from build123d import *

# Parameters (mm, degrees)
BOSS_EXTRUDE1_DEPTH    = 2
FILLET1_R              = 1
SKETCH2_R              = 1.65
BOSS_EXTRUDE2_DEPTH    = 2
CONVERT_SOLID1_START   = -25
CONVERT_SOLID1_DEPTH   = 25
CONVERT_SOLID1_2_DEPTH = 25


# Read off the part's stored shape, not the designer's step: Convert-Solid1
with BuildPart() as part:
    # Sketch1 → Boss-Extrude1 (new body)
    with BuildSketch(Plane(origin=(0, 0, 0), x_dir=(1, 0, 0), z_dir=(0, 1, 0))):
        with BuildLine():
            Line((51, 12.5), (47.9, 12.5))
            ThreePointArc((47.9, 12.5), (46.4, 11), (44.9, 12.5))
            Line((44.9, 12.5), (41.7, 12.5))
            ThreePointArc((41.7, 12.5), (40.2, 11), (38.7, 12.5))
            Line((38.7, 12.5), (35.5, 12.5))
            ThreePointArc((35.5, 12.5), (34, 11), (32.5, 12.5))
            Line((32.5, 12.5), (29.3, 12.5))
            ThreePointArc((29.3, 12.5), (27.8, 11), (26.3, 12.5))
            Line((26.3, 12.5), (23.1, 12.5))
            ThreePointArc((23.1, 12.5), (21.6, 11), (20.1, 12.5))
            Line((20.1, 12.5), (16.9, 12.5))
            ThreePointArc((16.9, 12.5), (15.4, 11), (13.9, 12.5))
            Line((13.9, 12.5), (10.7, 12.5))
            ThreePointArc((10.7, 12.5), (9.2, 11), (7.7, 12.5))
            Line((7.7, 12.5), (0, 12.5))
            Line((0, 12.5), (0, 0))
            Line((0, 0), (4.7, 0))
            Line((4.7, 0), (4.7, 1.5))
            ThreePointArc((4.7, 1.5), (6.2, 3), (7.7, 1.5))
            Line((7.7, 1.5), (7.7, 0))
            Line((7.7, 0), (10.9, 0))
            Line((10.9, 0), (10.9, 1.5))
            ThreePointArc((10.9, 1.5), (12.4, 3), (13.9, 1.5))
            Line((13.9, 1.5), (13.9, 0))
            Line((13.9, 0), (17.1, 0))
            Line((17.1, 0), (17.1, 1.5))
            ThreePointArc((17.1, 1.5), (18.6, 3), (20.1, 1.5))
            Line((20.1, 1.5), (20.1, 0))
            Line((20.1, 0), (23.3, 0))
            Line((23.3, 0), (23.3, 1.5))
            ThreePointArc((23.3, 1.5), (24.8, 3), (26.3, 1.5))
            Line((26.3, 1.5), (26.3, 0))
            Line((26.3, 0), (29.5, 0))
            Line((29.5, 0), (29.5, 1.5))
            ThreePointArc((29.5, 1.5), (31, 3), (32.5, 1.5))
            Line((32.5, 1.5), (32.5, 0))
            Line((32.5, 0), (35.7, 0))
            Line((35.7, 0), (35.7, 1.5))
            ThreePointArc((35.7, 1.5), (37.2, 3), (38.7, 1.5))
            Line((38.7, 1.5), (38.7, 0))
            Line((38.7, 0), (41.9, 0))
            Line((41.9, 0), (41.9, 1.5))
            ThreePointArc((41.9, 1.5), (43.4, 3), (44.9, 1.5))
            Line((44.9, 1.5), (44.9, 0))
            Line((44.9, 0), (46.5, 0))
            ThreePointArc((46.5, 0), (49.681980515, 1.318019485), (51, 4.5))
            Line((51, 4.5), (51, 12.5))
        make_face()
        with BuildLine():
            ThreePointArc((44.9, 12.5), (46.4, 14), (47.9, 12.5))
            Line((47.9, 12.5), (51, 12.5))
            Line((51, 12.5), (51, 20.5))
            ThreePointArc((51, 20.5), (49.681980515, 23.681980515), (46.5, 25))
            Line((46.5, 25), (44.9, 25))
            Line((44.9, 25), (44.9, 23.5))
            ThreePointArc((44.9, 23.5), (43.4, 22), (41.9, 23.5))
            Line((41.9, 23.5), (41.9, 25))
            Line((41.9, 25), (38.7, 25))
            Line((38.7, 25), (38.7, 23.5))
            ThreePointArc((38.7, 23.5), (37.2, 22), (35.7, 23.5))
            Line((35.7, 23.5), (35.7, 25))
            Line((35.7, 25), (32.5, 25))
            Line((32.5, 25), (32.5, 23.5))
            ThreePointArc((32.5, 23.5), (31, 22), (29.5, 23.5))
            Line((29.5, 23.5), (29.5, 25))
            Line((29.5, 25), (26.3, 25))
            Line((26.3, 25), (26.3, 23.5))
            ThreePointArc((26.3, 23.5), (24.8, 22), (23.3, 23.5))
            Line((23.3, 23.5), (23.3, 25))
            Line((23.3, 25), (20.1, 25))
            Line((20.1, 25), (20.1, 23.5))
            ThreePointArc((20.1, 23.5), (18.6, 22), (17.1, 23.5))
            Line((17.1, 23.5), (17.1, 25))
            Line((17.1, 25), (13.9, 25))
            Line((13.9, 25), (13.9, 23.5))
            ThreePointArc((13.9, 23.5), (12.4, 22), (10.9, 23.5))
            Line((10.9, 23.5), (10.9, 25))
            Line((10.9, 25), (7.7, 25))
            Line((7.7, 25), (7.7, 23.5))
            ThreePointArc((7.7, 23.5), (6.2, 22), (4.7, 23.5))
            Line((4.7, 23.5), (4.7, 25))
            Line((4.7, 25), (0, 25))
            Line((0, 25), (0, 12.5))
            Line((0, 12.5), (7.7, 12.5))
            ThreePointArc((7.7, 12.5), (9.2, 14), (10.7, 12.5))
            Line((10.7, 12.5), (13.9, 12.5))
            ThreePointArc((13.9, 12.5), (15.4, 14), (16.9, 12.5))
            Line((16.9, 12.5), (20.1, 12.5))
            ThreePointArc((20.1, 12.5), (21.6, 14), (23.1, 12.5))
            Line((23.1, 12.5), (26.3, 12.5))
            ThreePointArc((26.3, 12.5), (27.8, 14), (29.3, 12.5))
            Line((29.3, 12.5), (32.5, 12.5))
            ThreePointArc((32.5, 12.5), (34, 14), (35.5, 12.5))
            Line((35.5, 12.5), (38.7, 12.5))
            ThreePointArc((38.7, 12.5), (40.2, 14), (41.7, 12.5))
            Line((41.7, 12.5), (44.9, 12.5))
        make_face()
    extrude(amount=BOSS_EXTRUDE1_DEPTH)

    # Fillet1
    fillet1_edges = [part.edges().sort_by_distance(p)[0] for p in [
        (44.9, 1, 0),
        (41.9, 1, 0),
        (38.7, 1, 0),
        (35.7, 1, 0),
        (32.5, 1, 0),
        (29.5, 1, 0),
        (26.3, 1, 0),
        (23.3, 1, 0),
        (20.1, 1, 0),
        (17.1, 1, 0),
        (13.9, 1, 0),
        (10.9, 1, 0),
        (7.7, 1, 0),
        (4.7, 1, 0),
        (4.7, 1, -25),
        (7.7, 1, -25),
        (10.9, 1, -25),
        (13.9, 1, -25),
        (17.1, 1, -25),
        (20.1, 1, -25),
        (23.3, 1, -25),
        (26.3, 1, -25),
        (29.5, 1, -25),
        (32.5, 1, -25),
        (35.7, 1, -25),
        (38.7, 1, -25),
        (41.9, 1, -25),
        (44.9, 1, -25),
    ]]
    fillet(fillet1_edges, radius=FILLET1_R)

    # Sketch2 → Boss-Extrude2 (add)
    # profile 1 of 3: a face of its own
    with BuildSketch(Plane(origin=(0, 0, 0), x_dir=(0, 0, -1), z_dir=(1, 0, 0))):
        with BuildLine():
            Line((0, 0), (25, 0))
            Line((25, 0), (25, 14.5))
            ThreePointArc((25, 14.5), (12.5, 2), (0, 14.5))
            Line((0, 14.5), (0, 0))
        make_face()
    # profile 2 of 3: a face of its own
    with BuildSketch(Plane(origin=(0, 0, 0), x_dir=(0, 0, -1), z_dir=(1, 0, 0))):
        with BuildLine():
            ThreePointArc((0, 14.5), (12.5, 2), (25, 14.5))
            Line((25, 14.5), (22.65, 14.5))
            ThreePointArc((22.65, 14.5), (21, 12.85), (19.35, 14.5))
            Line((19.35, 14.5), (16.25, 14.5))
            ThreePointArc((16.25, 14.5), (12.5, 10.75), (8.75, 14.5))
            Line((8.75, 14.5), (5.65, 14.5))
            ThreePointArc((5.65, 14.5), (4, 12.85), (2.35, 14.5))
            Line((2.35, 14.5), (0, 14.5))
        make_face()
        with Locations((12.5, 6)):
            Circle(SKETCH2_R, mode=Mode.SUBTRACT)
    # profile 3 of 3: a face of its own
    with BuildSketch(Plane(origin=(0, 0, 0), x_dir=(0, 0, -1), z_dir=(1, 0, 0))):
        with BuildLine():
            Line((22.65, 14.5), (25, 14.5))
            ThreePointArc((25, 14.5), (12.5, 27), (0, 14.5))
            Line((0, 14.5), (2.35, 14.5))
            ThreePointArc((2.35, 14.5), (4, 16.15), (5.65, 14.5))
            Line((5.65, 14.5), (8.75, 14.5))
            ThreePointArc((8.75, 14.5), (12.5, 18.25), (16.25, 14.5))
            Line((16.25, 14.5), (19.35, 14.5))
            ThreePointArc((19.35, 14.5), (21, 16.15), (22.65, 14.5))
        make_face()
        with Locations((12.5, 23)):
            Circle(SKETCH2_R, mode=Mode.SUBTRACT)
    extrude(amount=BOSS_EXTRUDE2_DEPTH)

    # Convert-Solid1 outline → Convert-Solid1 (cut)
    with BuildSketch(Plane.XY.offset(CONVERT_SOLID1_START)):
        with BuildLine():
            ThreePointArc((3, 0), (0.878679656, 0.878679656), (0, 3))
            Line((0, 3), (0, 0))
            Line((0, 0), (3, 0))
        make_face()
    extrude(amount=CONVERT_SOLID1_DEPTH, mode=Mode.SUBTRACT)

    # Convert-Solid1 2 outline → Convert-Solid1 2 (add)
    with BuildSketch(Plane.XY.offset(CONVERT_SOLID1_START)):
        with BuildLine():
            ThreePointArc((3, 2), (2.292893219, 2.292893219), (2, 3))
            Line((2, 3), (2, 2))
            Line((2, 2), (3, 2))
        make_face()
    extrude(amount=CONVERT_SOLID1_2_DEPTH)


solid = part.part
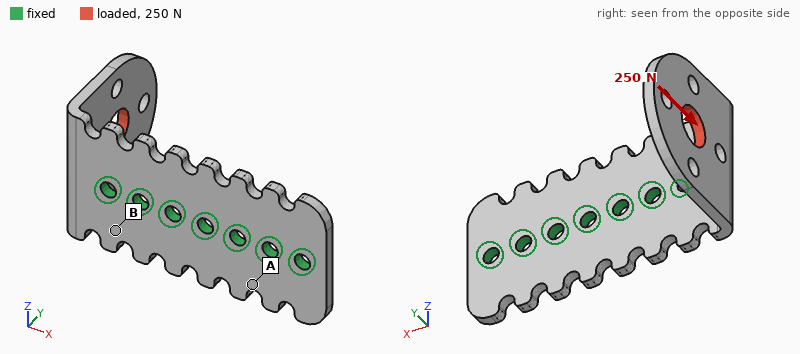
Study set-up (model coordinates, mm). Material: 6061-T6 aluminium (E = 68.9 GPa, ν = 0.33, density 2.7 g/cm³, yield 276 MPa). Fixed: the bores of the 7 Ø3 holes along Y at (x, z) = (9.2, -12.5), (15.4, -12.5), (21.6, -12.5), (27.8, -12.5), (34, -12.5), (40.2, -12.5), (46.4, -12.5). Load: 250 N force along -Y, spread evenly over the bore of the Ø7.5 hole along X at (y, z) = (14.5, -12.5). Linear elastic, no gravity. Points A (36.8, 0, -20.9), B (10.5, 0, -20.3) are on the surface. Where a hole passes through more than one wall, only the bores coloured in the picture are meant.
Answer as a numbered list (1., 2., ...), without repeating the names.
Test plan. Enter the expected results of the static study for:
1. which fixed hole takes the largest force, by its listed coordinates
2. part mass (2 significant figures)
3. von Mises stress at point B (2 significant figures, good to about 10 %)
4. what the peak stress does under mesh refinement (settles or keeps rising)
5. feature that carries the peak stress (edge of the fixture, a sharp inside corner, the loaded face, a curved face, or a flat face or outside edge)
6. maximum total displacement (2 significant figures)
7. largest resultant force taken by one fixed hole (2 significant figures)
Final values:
1. (9.2, -12.5)
2. 8.4 g
3. 45 MPa
4. keeps rising
5. edge of the fixture
6. 0.24 mm
7. 340 N
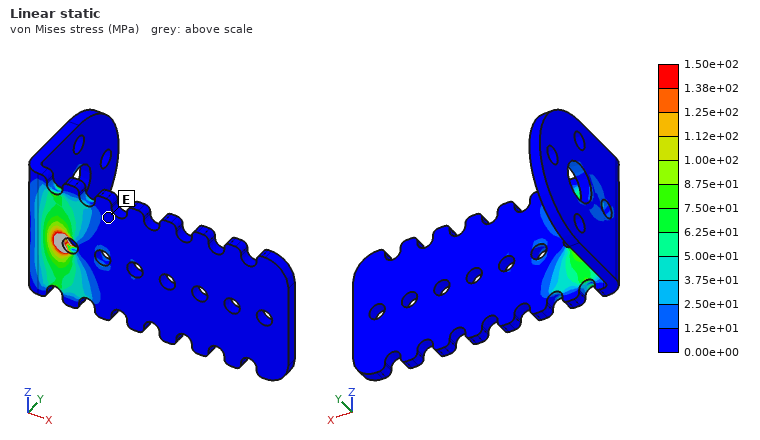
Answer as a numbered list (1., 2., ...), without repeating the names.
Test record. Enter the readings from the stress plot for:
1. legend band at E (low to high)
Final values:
1. 0.00e+00 to 1.25e+01 MPa
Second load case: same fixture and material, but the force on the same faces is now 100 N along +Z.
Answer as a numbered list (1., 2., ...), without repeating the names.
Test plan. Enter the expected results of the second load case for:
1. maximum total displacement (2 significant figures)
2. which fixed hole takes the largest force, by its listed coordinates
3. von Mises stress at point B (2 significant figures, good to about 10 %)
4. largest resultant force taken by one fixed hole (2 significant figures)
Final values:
1. 0.17 mm
2. (9.2, -12.5)
3. 42 MPa
4. 130 N
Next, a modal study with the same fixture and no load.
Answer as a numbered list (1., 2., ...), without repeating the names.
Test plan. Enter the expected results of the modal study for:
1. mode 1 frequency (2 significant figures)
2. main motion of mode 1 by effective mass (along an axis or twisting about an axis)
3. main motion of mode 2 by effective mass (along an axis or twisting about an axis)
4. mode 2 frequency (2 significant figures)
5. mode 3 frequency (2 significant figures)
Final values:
1. 1900 Hz
2. along X
3. along Z
4. 2800 Hz
5. 6500 Hz
